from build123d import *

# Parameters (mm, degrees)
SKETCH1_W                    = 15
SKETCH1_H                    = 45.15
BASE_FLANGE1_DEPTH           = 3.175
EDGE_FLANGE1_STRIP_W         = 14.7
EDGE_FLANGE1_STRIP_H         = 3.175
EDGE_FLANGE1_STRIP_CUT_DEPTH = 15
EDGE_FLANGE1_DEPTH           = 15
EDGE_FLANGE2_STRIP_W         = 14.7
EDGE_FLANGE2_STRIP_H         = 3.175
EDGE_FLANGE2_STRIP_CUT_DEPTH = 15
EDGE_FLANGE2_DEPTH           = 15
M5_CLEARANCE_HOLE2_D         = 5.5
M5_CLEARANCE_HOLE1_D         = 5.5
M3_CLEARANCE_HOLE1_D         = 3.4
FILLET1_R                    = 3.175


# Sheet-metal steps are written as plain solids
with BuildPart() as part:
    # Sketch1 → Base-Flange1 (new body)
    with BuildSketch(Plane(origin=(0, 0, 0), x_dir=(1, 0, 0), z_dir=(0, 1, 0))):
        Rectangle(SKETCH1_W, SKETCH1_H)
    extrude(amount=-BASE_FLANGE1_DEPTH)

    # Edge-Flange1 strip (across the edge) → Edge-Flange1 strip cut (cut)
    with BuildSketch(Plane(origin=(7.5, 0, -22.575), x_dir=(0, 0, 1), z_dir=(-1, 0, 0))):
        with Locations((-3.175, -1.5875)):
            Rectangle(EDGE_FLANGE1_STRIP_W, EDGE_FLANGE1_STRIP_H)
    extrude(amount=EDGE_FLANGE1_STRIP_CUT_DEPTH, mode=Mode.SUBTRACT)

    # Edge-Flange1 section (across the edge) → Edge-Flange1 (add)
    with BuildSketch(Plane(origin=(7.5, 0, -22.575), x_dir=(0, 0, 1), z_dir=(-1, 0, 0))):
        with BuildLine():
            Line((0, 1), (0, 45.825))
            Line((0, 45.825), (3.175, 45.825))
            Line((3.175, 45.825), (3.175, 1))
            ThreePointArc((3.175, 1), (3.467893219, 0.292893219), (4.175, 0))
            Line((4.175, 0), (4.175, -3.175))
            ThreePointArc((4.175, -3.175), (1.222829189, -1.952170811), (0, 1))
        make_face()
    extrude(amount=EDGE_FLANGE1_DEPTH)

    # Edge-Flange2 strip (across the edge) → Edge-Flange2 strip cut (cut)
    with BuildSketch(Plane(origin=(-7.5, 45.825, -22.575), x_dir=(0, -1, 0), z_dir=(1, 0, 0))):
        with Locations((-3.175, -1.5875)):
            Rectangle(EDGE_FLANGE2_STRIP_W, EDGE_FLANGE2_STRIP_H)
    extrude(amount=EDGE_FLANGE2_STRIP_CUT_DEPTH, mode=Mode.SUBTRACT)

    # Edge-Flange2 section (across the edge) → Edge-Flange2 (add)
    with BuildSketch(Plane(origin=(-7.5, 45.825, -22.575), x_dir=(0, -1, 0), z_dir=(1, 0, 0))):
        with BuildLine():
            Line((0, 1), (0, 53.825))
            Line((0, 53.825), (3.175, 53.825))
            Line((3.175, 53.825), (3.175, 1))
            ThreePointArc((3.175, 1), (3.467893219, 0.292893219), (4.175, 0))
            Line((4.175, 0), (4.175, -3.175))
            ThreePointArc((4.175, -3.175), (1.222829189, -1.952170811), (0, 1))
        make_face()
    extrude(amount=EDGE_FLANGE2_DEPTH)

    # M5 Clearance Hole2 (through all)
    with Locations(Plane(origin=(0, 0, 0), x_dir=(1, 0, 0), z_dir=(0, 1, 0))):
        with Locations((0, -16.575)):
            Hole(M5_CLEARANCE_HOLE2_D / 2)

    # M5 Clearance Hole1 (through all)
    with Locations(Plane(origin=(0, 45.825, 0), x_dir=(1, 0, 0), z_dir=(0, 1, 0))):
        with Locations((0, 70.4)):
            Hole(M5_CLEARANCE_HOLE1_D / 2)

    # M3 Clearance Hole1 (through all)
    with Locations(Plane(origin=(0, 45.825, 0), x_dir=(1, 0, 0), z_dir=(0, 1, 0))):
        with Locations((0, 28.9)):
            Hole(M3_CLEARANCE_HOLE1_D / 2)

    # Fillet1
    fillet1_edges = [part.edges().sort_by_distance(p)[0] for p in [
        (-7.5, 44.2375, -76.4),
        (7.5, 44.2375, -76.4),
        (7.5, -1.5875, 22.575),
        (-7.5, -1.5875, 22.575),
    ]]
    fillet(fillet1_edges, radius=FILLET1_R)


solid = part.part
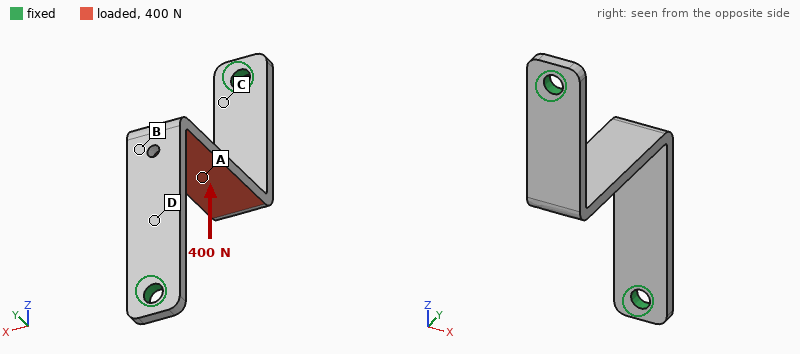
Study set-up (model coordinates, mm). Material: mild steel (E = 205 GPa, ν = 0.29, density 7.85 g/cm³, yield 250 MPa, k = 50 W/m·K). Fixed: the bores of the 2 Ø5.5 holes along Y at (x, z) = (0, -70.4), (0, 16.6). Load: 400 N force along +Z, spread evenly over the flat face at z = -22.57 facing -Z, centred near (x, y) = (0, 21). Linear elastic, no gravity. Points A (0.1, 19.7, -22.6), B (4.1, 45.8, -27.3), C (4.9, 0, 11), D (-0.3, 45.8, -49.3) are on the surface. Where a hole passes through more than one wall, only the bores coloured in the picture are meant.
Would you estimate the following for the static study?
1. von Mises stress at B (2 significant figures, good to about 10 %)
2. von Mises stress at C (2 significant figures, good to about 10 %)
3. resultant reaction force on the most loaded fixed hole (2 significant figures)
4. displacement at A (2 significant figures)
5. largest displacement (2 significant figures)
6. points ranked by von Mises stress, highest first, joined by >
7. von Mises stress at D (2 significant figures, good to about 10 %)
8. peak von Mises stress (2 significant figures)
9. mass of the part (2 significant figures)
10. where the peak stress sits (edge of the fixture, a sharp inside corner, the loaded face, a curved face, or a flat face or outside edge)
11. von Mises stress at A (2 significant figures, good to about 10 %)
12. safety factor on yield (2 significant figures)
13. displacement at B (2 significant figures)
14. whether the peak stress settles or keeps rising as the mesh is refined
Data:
25 MPa
34 MPa
200 N
77 µm
78 µm
A > C > B > D
14 MPa
76 MPa
52 g
a flat face or outside edge
73 MPa
3.3
43 µm
settles
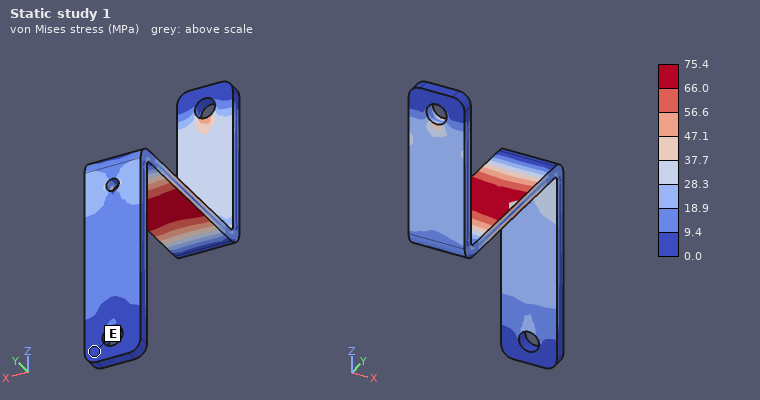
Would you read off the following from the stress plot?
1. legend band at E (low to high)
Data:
0.0 to 9.4 MPa
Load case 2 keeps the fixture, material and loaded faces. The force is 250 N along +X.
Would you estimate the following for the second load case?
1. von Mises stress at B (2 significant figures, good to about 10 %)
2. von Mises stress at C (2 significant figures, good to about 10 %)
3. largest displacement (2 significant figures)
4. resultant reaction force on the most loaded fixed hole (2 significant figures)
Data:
6.5 MPa
22 MPa
33 µm
130 N
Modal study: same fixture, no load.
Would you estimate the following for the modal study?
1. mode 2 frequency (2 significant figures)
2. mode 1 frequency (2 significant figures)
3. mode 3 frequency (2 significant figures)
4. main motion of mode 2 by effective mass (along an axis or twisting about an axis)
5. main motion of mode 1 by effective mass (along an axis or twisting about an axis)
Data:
2900 Hz
1200 Hz
4600 Hz
along X
along Y
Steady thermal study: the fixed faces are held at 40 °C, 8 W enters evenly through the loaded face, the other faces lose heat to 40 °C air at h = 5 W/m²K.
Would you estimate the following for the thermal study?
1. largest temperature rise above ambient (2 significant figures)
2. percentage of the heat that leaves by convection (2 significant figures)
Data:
83 K
11 %
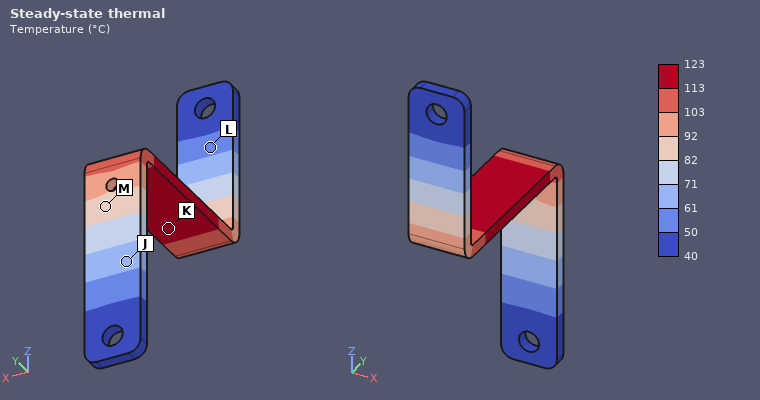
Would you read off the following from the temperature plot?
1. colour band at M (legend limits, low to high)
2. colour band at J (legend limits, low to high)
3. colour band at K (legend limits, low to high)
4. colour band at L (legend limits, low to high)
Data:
82 to 92 °C
61 to 71 °C
113 to 123 °C
50 to 61 °C
